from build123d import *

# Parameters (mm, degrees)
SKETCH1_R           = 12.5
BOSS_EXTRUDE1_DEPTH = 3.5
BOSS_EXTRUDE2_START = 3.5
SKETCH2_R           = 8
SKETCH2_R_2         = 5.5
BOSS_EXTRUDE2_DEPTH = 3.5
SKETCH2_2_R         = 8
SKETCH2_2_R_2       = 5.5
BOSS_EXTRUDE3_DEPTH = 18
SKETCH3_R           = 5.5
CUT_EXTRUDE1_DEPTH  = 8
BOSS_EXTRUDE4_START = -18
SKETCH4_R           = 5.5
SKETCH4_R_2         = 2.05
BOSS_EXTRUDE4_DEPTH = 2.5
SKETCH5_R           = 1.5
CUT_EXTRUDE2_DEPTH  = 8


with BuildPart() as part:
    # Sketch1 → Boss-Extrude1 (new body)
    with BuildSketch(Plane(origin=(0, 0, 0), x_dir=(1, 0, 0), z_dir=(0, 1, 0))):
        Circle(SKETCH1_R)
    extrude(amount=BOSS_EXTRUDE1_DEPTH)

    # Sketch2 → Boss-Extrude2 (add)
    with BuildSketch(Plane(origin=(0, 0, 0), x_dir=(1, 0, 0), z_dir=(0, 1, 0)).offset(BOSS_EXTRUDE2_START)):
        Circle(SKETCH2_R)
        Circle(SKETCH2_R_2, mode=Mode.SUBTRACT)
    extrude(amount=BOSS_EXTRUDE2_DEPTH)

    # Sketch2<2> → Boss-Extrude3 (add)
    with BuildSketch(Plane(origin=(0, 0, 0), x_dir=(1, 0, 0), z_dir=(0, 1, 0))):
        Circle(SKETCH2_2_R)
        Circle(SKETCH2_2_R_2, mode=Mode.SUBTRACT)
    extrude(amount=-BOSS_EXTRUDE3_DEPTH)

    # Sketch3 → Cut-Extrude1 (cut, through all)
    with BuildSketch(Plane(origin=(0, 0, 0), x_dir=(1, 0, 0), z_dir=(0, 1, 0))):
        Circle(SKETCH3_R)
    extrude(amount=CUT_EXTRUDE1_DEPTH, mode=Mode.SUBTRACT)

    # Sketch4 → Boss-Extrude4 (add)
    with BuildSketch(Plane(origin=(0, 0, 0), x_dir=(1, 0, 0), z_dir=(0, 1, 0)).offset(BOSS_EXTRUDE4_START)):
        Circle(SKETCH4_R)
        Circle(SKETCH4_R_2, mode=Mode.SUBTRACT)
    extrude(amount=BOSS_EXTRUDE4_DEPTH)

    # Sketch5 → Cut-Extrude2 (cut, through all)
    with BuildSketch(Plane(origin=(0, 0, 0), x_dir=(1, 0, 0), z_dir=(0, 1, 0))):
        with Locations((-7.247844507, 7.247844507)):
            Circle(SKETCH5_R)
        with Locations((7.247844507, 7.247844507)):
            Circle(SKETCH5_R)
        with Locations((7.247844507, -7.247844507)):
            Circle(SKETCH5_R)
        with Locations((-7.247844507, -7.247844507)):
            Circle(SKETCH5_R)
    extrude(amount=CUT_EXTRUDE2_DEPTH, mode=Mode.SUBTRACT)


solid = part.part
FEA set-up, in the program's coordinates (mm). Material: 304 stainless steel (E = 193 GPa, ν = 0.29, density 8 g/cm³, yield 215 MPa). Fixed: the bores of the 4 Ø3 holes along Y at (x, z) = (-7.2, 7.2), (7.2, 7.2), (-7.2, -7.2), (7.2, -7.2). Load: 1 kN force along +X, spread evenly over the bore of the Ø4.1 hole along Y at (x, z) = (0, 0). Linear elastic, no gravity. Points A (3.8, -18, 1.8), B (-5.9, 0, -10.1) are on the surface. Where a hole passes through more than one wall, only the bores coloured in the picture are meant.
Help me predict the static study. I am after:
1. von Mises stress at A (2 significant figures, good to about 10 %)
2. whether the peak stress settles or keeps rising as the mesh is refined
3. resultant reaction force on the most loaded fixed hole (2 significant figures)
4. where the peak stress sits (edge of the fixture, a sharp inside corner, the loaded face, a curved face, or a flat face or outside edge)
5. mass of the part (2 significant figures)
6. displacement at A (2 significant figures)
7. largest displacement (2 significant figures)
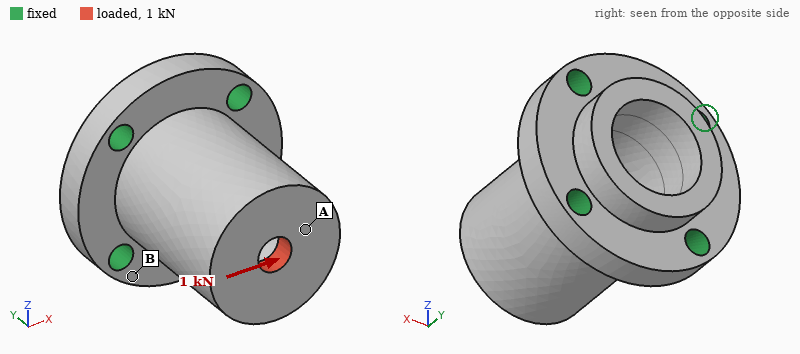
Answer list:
26 MPa
keeps rising
720 N
edge of the fixture
30 g
12 µm
13 µm
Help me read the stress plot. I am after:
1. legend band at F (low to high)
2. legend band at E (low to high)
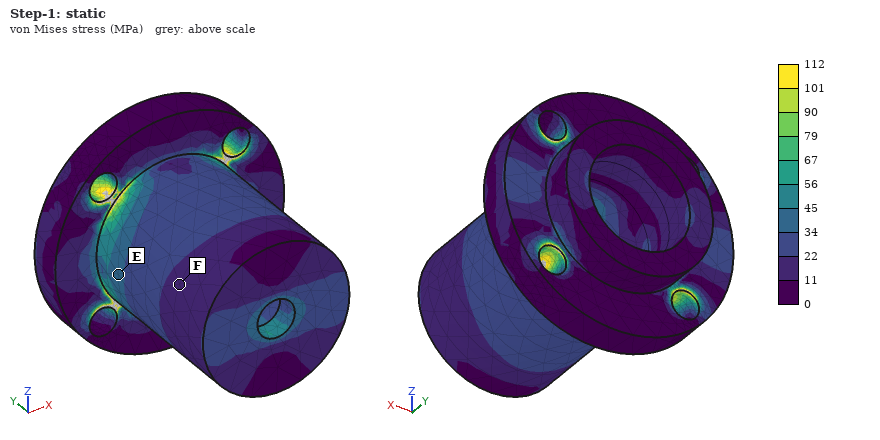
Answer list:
11 to 22 MPa
34 to 45 MPa
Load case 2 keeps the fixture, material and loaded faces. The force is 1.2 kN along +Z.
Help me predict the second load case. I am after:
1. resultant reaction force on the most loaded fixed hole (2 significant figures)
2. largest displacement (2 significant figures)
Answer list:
870 N
15 µm
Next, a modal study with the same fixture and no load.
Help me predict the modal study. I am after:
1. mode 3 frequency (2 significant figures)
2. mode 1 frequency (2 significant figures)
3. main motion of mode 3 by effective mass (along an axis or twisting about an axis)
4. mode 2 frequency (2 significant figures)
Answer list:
37 kHz
17 kHz
twisting about Y
17 kHz
